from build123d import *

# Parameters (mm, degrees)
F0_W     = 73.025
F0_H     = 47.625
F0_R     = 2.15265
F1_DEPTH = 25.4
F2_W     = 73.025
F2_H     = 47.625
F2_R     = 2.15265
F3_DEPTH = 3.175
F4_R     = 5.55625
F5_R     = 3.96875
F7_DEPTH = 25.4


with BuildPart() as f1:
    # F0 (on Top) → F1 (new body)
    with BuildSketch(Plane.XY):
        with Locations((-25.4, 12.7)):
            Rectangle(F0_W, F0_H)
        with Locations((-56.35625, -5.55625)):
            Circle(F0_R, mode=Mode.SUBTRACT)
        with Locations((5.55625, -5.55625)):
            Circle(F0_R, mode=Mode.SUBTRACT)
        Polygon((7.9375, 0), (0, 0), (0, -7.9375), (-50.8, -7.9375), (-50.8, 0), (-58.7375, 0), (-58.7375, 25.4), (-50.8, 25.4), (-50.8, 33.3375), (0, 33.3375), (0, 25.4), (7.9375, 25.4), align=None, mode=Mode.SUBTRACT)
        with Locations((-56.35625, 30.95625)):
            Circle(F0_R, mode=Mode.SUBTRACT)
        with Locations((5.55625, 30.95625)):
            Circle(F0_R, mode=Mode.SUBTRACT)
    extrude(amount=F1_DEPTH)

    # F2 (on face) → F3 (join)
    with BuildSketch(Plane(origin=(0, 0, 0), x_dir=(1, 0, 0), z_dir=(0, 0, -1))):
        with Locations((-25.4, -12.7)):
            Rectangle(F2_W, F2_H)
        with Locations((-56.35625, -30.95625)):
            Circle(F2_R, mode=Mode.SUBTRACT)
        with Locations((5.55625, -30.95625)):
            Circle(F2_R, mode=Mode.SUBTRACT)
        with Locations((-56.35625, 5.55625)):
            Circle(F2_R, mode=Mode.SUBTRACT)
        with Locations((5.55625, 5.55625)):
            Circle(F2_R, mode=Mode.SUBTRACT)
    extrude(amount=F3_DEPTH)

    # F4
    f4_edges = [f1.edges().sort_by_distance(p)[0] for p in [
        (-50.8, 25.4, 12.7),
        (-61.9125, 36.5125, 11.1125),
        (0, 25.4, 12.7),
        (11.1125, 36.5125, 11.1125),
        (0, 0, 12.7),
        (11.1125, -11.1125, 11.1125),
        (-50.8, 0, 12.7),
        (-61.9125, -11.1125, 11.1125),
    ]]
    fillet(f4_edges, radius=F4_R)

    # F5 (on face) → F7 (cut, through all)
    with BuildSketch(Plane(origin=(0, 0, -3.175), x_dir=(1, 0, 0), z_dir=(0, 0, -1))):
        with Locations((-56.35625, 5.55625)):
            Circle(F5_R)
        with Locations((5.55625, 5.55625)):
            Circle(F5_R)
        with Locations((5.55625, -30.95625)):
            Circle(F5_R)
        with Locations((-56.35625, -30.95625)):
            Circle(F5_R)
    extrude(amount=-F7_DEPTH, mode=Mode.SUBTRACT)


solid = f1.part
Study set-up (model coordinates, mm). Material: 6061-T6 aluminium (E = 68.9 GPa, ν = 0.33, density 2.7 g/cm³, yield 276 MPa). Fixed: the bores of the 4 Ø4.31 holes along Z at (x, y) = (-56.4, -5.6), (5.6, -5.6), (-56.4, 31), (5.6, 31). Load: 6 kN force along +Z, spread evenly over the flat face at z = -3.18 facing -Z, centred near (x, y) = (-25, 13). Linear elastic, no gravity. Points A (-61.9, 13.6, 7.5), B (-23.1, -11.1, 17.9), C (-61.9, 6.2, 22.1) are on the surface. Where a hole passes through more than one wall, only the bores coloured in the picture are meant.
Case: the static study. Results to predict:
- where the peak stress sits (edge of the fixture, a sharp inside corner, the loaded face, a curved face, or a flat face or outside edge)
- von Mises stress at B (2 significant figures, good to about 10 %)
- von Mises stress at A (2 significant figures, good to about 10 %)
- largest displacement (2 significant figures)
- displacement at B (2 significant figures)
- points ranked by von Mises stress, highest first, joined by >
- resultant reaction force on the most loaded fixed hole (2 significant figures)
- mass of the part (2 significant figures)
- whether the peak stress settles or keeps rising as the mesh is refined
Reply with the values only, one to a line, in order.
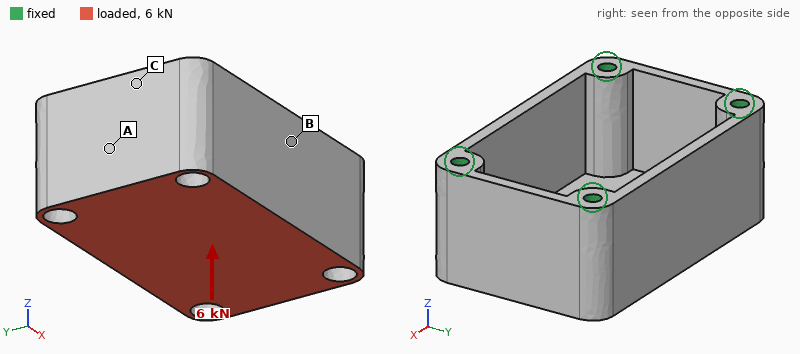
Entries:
edge of the fixture
29 MPa
16 MPa
0.15 mm
0.048 mm
B > A > C
1.6 kN
79 g
keeps rising
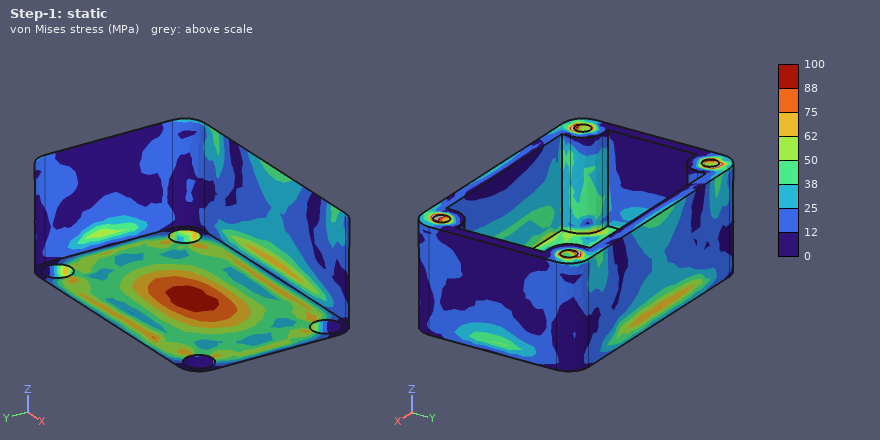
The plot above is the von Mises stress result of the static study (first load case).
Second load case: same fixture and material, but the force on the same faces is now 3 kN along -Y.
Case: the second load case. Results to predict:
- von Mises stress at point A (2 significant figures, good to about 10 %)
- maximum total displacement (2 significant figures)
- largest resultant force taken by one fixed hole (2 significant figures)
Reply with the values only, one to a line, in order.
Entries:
23 MPa
33 µm
1.3 kN
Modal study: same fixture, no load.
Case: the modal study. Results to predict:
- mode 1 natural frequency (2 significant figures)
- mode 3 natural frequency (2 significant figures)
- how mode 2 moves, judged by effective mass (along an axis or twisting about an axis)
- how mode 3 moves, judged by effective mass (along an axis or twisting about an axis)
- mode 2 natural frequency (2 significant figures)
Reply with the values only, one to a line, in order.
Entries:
6200 Hz
8500 Hz
along Y
along Y
6600 Hz
